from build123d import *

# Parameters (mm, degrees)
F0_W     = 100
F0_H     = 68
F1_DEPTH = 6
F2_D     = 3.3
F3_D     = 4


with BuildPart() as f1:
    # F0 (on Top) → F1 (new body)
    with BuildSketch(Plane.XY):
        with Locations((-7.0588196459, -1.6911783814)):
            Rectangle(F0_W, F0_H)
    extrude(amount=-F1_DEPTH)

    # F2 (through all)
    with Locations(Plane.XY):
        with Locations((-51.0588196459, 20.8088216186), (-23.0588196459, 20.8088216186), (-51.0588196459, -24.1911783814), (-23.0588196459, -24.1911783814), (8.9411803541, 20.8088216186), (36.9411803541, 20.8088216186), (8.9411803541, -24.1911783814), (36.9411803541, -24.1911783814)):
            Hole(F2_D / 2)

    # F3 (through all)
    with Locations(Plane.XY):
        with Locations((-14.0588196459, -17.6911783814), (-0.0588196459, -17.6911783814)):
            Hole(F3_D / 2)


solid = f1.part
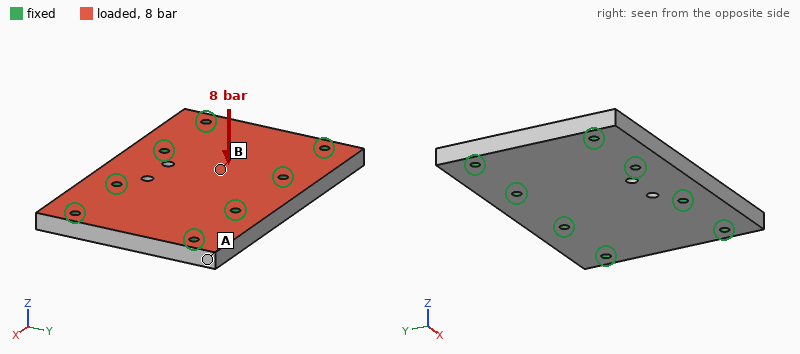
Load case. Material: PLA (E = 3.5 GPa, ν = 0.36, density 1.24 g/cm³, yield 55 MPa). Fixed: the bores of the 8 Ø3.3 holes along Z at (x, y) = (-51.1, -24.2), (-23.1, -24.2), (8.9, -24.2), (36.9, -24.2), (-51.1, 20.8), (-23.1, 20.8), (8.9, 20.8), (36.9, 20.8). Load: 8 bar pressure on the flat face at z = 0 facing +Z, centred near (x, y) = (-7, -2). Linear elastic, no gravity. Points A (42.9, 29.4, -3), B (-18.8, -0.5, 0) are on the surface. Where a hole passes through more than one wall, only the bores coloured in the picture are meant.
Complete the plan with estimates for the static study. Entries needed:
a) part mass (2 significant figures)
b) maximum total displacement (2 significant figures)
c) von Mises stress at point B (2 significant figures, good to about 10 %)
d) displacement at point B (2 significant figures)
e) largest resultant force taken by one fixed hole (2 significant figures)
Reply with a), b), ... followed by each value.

a) 50 g
b) 0.23 mm
c) 11 MPa
d) 0.22 mm
e) 830 N
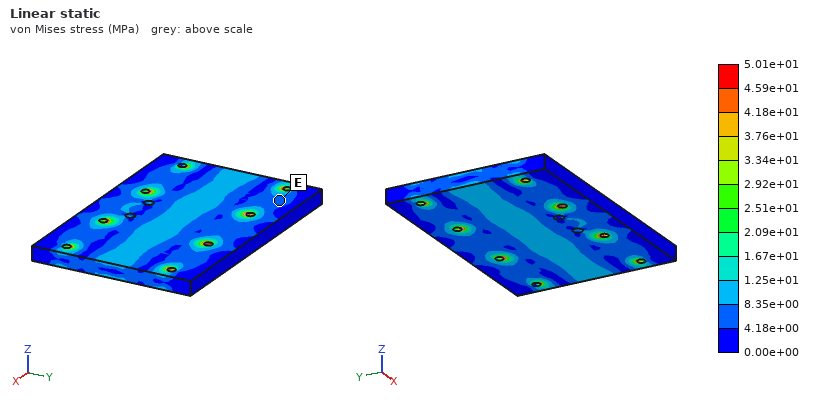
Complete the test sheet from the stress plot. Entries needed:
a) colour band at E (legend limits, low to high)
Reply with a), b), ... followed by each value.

a) 4.18e+00 to 8.35e+00 MPa
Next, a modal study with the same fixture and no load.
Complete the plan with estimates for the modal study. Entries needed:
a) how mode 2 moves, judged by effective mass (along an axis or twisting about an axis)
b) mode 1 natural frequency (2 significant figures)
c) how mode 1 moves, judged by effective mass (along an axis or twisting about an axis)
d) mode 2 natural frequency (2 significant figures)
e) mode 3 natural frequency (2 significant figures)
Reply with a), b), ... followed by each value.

a) twisting about Y
b) 3800 Hz
c) along Z
d) 4300 Hz
e) 4900 Hz
